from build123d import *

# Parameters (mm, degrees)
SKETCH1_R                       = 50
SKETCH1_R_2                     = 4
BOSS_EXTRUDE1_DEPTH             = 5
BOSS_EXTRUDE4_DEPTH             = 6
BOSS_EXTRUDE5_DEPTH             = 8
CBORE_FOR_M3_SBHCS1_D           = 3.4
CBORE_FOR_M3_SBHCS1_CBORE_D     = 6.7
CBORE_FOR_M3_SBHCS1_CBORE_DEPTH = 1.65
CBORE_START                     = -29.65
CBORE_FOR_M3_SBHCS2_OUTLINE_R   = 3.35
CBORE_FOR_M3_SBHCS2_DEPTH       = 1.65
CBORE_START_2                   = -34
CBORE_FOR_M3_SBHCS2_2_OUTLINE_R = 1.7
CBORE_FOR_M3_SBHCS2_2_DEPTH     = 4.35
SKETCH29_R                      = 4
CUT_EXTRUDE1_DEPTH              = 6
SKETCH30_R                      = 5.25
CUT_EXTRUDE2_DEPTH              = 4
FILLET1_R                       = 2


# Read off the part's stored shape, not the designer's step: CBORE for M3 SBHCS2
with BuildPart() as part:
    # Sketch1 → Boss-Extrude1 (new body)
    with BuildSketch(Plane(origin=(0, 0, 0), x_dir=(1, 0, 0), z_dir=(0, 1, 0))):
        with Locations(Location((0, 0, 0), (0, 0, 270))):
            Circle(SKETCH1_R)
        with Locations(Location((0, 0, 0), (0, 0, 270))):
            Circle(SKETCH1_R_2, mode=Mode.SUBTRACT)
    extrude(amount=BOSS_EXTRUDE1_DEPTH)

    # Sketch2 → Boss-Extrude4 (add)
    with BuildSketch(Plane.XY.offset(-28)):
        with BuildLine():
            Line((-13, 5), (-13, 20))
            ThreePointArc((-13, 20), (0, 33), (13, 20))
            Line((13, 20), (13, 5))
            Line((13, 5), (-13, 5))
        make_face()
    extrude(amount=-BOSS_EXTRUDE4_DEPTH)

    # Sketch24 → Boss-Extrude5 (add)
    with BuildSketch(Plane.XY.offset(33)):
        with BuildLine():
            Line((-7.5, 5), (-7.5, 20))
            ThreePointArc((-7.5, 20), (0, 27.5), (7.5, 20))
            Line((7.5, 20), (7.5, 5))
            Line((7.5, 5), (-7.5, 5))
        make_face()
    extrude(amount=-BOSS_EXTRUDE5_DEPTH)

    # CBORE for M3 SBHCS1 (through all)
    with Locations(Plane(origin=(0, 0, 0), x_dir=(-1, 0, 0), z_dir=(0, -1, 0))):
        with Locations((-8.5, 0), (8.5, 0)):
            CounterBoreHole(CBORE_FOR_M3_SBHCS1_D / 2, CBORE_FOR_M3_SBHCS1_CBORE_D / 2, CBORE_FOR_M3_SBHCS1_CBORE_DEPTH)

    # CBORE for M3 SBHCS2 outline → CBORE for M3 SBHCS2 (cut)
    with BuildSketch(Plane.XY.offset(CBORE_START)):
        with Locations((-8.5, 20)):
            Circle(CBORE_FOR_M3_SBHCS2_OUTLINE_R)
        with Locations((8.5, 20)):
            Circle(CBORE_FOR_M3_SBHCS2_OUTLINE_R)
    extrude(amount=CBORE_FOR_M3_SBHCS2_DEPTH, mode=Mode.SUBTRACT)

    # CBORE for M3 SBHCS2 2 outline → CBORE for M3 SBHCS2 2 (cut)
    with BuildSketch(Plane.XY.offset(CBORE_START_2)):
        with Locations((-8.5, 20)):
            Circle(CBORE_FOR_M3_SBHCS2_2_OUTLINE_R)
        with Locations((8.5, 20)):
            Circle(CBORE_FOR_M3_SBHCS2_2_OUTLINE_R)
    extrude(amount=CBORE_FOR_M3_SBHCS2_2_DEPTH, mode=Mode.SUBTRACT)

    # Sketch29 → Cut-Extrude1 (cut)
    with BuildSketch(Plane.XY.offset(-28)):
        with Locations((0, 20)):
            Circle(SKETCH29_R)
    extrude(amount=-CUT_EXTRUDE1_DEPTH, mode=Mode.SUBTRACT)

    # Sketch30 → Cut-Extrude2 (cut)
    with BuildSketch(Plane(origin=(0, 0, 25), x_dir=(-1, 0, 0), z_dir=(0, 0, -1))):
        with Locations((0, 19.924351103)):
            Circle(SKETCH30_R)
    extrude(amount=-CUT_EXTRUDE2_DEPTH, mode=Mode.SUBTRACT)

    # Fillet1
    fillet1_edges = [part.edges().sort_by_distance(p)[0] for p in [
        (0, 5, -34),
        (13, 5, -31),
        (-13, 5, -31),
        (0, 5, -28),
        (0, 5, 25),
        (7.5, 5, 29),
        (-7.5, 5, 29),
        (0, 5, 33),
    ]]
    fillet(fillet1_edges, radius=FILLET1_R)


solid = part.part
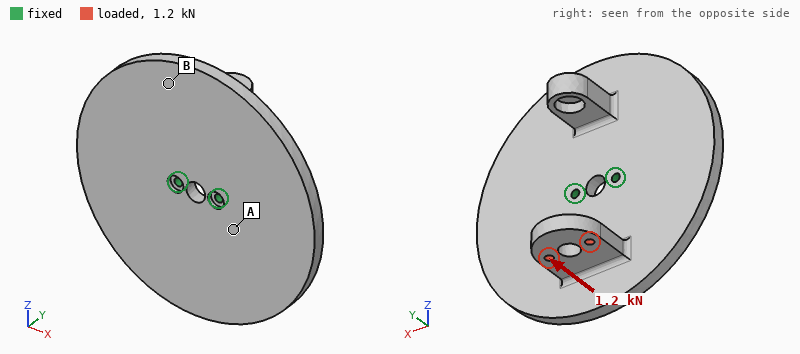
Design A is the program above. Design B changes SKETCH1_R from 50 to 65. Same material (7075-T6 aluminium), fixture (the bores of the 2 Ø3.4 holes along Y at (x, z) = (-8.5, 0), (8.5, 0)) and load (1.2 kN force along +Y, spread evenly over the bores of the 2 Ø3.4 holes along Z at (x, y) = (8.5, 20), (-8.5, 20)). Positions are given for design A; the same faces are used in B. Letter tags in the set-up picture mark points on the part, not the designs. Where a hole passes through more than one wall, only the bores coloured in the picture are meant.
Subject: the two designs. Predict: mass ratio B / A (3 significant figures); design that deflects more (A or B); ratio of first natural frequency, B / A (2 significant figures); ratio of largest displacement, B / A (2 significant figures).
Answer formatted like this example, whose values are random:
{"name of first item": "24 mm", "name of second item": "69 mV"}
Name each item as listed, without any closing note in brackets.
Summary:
{"mass ratio B / A": "1.61", "design that deflects more": "B", "ratio of first natural frequency, B / A": "0.62", "ratio of largest displacement, B / A": "1.2"}
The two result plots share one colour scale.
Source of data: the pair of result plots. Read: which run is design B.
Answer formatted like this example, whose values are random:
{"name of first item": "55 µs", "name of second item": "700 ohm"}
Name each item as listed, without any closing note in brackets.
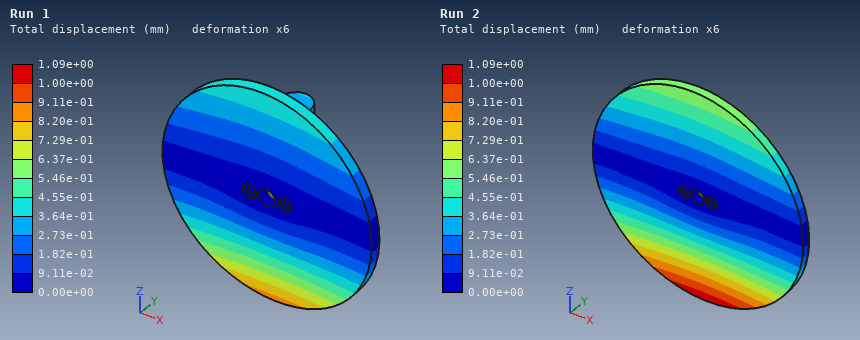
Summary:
{"which run is design B": "Run 2"}
